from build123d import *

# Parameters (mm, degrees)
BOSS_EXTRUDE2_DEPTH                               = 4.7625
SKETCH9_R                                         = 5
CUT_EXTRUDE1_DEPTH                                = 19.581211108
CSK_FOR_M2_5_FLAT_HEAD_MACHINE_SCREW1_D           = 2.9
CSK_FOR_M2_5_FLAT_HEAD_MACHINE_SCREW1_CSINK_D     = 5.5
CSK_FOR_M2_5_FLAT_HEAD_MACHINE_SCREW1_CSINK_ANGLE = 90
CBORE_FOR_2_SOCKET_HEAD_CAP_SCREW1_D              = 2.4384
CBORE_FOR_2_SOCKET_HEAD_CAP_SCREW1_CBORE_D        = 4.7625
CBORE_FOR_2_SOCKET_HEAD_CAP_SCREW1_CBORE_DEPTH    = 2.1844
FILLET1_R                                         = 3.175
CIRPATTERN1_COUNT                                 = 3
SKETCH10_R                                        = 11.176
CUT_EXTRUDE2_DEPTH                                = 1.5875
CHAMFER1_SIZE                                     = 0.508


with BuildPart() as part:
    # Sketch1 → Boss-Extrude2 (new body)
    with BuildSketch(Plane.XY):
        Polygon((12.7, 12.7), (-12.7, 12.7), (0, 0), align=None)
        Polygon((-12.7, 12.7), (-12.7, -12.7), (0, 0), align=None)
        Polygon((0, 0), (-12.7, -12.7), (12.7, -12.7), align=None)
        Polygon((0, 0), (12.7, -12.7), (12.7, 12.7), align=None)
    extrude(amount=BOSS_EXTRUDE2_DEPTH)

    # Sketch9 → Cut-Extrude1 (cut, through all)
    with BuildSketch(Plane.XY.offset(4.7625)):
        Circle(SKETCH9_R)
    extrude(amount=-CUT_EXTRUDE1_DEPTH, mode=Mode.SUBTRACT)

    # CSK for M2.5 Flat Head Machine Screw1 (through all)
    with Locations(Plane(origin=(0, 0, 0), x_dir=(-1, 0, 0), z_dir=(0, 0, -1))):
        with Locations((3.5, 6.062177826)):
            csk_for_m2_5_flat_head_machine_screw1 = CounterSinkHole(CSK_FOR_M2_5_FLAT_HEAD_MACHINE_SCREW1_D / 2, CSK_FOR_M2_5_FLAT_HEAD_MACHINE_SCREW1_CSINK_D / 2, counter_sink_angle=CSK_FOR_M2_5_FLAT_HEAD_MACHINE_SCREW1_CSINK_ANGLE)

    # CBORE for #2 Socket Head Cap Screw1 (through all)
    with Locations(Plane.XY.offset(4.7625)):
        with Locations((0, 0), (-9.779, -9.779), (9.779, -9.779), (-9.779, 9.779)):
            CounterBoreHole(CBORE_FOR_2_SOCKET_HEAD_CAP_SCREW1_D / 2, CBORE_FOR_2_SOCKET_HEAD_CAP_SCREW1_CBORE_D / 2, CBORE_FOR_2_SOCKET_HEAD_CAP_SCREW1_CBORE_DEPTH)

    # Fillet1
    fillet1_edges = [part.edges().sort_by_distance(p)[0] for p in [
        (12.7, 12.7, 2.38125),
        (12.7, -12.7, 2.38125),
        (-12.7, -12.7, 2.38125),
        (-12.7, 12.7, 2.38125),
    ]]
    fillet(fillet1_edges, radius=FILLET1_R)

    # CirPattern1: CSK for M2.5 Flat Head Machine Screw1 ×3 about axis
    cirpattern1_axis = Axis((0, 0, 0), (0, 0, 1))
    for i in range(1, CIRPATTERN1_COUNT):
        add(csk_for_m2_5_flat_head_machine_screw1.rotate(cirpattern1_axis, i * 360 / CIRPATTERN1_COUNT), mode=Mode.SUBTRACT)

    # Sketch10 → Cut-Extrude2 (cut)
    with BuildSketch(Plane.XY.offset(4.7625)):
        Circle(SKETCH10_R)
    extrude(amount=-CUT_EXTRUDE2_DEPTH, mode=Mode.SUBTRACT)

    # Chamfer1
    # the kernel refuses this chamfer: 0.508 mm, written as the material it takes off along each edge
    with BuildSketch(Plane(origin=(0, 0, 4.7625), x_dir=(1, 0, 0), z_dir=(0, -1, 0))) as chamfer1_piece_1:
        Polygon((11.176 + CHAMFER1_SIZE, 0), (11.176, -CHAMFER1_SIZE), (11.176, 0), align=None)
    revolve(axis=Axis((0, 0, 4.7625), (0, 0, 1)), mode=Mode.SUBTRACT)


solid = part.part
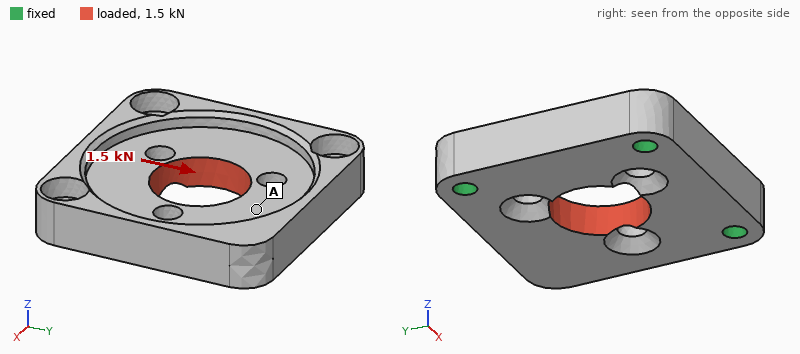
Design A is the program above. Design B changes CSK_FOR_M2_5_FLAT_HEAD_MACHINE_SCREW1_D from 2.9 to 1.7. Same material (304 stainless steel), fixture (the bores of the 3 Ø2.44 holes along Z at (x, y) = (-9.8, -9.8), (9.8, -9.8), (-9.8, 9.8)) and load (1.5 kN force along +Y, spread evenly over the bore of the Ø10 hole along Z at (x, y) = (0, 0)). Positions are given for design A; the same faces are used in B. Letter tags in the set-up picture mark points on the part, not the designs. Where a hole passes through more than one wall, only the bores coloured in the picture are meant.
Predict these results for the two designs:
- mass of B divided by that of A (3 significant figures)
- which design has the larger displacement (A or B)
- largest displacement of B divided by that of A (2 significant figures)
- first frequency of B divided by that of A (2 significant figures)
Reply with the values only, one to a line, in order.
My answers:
1.01
A
0.85
1.0
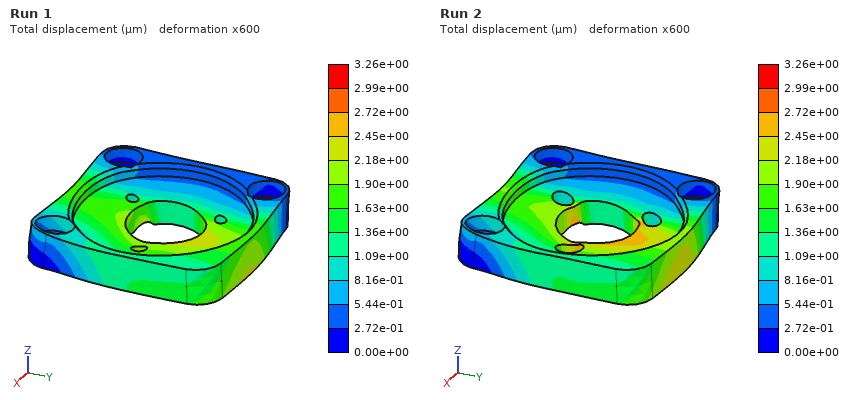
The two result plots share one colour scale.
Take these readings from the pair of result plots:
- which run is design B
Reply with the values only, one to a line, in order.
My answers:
Run 1
